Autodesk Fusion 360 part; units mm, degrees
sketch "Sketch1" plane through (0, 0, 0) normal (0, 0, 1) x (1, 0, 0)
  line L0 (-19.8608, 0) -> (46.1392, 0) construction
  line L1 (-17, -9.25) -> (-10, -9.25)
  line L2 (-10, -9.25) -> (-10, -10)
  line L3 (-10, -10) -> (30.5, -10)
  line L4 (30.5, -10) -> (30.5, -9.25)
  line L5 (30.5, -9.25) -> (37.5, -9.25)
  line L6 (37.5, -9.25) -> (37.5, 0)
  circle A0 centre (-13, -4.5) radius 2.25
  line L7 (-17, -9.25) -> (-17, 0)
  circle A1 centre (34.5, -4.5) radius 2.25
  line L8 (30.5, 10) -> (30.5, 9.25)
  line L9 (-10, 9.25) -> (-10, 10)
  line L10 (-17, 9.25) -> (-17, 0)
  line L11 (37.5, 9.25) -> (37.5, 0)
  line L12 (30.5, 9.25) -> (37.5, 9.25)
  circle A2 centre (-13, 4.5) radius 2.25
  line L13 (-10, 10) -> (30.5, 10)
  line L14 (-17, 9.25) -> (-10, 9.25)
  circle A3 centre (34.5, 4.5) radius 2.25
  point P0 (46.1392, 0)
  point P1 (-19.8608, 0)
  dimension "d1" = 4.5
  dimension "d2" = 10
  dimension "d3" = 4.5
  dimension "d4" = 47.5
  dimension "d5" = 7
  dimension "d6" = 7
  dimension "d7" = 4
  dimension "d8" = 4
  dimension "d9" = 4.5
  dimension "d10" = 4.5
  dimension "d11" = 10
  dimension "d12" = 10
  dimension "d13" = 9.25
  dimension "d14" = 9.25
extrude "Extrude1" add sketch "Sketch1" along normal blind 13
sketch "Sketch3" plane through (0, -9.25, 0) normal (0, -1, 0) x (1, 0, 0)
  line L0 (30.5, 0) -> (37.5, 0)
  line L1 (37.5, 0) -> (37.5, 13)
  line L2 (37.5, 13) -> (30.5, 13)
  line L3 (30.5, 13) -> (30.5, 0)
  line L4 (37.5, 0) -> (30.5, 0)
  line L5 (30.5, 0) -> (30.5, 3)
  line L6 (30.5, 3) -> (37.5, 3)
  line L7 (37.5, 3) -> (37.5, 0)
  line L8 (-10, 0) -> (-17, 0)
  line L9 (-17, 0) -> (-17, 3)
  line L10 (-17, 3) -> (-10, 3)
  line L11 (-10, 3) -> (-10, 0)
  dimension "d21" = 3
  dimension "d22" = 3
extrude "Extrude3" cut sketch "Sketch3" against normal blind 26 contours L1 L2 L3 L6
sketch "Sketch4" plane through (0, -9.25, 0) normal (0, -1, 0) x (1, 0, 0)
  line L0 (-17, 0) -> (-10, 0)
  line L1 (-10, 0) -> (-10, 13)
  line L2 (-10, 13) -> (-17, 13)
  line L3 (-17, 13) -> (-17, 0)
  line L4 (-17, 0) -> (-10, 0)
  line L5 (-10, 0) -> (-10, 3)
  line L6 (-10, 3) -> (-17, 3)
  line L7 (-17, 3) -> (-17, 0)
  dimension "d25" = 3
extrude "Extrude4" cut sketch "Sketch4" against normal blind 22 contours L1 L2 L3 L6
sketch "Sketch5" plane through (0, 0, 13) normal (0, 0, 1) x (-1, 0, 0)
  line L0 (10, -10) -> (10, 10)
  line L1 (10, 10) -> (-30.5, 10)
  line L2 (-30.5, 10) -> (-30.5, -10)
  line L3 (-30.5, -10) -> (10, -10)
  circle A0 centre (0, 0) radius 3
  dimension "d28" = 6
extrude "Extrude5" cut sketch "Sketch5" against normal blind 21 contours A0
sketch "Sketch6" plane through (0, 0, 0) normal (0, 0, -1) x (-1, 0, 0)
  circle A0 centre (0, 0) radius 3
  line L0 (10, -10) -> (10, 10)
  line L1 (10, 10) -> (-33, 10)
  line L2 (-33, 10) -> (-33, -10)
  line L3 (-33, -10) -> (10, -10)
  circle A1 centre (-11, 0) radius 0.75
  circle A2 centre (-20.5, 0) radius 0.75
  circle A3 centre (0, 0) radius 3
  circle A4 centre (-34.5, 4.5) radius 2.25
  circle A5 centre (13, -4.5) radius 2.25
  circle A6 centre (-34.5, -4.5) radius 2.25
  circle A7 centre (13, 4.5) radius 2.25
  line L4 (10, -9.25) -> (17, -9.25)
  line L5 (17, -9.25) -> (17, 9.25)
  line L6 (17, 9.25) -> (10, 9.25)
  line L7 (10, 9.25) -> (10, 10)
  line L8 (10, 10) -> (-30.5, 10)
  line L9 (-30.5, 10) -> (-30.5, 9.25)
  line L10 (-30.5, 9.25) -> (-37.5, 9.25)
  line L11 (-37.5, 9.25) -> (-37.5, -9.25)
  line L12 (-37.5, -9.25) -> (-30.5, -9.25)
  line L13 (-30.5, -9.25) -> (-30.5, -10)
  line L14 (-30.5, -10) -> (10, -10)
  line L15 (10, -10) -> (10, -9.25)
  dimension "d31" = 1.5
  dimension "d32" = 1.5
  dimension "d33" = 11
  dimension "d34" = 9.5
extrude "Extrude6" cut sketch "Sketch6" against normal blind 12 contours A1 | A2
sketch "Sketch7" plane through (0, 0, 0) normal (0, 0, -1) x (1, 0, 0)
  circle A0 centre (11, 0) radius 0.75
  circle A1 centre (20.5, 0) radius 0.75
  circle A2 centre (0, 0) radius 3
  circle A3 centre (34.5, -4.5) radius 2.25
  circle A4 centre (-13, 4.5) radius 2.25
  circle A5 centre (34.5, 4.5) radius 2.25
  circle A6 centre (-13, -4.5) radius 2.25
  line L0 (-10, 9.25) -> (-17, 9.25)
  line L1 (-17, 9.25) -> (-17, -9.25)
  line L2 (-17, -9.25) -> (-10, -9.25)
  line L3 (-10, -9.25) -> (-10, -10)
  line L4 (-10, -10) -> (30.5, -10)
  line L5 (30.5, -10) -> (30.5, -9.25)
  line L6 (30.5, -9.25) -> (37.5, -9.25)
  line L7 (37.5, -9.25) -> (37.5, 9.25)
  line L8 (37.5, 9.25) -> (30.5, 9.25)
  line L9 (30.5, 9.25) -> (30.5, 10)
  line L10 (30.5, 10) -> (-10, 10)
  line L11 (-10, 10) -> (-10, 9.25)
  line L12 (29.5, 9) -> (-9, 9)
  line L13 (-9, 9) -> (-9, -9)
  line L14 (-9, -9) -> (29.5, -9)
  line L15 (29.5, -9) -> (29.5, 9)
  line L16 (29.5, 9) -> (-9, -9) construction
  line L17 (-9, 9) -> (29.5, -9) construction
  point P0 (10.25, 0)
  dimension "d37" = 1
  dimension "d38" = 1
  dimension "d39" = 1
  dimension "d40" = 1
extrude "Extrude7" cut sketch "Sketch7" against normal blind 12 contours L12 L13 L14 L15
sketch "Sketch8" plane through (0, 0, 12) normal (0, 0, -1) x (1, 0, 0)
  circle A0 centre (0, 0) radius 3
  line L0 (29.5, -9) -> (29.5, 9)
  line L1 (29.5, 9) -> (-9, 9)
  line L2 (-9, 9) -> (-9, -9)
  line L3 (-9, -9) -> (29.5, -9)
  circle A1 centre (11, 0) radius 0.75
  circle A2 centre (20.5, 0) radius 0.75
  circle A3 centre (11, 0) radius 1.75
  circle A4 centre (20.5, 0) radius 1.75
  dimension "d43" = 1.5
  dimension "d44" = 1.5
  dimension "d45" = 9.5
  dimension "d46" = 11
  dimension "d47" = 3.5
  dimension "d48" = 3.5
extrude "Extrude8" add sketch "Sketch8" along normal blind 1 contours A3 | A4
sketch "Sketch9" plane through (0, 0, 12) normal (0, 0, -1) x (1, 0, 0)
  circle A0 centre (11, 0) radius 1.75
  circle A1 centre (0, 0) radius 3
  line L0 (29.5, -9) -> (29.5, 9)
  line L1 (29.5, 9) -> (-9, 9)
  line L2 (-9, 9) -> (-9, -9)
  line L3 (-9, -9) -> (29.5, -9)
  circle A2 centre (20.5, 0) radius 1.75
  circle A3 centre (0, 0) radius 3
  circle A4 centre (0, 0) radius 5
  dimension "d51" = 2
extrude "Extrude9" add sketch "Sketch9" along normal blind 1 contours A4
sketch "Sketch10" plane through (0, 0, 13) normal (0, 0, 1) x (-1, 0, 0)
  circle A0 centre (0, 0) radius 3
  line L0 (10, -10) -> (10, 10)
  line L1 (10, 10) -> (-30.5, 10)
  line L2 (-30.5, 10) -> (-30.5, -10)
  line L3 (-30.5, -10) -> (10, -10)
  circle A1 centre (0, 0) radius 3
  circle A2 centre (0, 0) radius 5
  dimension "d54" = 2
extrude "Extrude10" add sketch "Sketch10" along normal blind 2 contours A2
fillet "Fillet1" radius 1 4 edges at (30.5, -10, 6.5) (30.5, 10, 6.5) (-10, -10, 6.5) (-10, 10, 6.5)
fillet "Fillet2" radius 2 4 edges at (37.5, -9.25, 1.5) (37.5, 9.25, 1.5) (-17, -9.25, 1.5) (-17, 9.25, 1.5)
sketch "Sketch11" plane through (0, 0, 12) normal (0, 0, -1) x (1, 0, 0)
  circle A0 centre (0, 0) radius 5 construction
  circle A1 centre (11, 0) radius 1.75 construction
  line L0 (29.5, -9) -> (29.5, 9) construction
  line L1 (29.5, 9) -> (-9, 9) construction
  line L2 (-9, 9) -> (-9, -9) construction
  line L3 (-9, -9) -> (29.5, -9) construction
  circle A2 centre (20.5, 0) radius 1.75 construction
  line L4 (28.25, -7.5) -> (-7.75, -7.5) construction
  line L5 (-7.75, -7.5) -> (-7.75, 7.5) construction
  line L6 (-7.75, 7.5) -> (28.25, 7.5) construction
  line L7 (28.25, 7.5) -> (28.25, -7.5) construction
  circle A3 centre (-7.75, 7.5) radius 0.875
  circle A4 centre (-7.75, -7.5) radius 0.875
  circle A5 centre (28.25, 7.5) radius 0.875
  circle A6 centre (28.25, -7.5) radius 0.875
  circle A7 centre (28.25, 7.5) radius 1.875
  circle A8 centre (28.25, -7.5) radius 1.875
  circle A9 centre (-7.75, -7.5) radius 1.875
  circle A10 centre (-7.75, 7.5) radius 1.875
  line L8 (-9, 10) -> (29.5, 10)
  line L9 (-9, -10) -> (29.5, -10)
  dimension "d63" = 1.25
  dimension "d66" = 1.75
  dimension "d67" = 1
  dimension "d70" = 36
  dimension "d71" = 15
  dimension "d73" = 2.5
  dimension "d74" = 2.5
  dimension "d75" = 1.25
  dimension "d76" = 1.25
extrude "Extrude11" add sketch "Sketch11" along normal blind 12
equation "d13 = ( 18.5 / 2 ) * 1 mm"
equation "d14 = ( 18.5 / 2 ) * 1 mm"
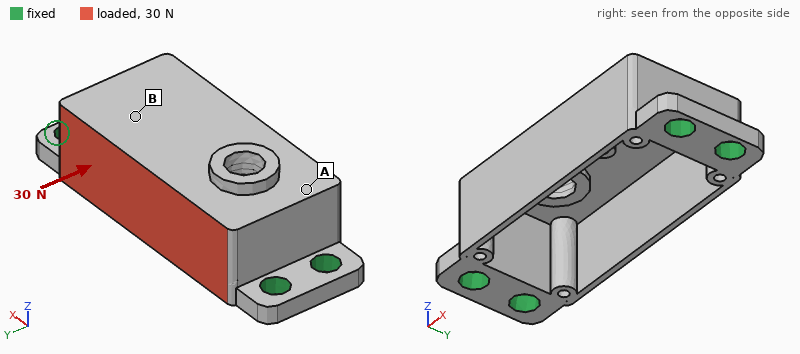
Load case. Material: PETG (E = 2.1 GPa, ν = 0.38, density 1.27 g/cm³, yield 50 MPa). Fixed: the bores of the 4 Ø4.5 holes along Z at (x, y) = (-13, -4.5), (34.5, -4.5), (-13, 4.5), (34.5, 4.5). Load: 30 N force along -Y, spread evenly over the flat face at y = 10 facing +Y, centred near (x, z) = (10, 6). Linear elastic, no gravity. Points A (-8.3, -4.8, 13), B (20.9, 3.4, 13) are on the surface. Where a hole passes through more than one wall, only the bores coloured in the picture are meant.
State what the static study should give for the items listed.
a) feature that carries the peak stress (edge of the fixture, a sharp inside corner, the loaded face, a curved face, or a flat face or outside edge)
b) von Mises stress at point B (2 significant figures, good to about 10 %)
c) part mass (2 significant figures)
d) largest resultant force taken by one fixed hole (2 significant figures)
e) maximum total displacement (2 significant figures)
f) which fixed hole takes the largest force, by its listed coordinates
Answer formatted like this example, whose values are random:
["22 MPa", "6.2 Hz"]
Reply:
["the loaded face", "1.8 MPa", "4.1 g", "12 N", "0.71 mm", "(-13, 4.5)"]
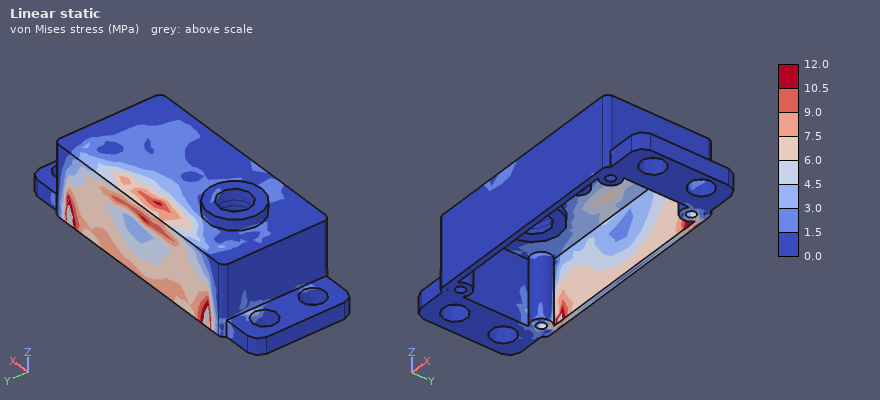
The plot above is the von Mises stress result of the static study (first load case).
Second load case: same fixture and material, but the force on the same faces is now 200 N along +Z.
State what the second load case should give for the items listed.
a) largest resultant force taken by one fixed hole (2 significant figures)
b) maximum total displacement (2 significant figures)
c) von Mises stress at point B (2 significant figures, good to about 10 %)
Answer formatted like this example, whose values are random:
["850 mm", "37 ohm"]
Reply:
["160 N", "0.63 mm", "4.6 MPa"]
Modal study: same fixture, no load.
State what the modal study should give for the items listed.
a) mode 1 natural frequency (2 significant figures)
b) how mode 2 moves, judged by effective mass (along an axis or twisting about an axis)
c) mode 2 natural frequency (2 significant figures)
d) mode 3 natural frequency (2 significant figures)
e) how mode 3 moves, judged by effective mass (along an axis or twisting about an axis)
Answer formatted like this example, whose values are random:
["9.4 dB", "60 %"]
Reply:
["1700 Hz", "along Y", "1800 Hz", "3200 Hz", "along Z"]
